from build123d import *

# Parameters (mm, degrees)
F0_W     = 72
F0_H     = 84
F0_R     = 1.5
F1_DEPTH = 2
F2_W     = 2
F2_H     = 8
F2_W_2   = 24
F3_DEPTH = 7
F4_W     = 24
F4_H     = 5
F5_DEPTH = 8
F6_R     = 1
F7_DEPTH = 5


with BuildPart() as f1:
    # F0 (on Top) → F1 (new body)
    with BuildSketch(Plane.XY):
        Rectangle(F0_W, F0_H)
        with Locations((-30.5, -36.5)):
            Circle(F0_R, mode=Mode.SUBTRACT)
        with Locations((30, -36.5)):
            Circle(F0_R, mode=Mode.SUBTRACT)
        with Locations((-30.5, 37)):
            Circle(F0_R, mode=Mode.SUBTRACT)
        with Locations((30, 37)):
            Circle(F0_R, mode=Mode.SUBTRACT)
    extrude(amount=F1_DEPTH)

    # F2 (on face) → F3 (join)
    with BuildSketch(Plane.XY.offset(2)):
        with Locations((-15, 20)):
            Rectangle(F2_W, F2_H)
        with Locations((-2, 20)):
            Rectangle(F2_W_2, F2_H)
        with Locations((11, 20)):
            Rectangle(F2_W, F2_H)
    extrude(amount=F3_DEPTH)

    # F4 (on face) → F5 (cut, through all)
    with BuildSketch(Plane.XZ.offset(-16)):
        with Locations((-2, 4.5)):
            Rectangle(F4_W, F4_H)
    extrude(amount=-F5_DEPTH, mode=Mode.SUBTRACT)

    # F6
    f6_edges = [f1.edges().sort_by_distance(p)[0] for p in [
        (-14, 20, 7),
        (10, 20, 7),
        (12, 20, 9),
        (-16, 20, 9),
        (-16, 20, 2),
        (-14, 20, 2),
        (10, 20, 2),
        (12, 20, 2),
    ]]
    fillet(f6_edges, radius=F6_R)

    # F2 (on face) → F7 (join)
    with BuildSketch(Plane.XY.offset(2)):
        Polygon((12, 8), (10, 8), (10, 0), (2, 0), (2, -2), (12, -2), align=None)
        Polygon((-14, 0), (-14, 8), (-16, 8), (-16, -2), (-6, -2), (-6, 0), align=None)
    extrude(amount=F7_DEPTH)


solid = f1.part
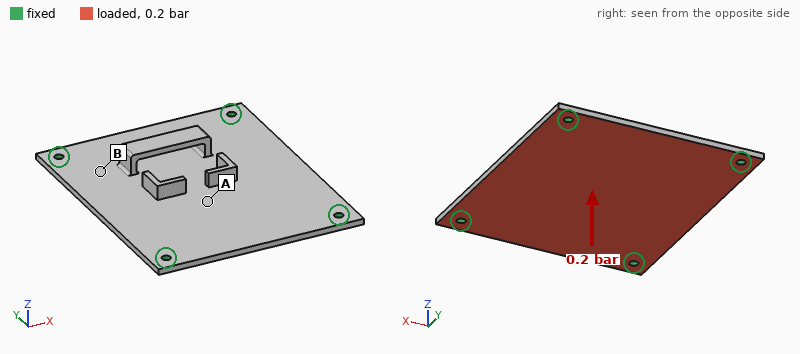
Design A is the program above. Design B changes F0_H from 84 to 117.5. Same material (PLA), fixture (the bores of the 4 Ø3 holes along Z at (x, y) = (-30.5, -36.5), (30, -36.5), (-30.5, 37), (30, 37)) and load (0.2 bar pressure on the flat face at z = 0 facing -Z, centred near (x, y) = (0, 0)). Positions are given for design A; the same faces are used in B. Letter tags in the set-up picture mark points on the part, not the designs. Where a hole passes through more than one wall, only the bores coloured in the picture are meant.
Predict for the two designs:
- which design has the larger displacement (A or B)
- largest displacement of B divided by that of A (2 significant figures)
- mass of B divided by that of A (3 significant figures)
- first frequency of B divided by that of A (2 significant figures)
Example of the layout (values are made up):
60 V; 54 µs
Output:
A; 0.87; 1.37; 1.0
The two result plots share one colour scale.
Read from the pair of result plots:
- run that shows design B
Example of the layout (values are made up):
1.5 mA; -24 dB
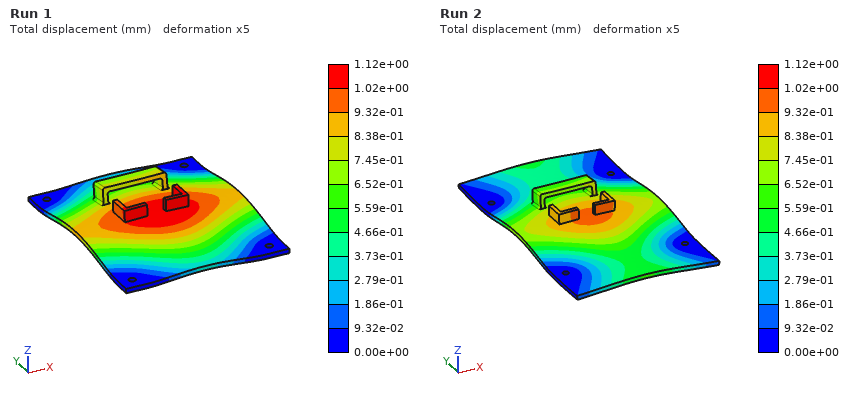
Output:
Run 2
